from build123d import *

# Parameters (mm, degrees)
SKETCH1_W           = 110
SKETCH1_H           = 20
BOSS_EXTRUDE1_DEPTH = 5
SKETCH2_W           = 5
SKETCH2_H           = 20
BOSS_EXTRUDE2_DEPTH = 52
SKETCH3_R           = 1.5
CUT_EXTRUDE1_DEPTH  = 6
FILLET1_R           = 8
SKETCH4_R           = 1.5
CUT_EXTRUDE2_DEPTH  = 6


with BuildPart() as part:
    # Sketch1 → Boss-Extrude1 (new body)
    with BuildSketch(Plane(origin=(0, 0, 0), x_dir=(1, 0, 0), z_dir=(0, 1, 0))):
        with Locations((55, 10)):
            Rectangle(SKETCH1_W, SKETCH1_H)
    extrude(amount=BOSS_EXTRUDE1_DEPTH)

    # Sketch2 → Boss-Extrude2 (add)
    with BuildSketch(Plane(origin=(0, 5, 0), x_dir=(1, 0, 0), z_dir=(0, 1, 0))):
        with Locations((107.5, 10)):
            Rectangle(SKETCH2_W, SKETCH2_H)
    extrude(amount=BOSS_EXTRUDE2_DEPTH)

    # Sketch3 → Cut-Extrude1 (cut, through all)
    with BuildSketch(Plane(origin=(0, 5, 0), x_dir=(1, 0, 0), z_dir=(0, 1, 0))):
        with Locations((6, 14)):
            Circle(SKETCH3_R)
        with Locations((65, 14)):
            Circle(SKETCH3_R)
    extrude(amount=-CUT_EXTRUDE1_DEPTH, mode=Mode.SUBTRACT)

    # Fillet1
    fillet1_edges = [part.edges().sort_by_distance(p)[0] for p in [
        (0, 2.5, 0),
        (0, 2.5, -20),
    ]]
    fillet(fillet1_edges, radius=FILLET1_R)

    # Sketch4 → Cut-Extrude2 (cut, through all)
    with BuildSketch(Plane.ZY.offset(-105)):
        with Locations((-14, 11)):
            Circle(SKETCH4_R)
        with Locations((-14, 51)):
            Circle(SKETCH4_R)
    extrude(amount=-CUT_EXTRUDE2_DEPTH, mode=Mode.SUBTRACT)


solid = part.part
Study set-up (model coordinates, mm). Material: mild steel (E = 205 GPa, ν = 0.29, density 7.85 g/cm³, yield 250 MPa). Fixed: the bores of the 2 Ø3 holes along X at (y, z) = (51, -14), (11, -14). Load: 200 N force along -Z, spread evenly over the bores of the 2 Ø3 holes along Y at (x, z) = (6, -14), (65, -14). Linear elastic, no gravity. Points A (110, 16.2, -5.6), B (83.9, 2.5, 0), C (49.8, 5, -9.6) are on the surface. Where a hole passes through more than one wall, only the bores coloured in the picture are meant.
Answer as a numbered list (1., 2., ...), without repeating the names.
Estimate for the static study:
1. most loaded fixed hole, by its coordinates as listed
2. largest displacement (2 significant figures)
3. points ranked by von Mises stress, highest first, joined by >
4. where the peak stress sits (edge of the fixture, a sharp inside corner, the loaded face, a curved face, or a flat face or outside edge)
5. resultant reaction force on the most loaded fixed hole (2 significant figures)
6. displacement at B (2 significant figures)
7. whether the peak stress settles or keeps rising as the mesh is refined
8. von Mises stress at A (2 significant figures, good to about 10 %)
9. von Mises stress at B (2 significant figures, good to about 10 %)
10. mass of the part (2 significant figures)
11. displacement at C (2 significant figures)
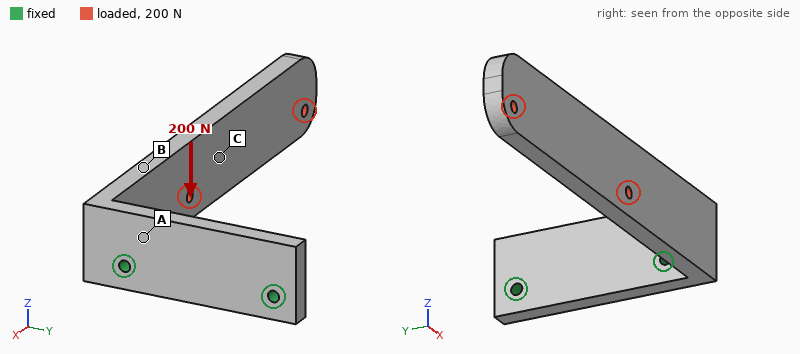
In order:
1. (11, -14)
2. 0.30 mm
3. A > B > C
4. edge of the fixture
5. 240 N
6. 0.067 mm
7. keeps rising
8. 56 MPa
9. 29 MPa
10. 120 g
11. 0.15 mm
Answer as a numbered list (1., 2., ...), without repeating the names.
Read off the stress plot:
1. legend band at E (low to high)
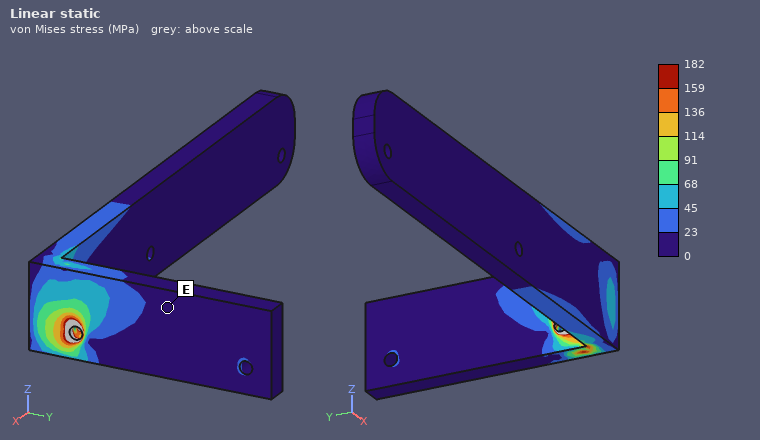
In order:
1. 0 to 23 MPa
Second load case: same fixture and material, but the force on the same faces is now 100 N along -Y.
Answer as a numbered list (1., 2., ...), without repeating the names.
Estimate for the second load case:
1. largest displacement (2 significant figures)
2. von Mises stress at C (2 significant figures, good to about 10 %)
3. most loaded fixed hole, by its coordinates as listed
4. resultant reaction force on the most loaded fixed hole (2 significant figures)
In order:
1. 0.69 mm
2. 27 MPa
3. (11, -14)
4. 110 N
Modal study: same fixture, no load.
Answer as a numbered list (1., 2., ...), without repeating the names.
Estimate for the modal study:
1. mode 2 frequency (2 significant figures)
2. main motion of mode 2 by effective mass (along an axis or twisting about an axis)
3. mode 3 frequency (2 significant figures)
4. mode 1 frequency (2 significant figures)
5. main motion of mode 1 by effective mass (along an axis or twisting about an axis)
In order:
1. 660 Hz
2. along Z
3. 2000 Hz
4. 320 Hz
5. along Y
